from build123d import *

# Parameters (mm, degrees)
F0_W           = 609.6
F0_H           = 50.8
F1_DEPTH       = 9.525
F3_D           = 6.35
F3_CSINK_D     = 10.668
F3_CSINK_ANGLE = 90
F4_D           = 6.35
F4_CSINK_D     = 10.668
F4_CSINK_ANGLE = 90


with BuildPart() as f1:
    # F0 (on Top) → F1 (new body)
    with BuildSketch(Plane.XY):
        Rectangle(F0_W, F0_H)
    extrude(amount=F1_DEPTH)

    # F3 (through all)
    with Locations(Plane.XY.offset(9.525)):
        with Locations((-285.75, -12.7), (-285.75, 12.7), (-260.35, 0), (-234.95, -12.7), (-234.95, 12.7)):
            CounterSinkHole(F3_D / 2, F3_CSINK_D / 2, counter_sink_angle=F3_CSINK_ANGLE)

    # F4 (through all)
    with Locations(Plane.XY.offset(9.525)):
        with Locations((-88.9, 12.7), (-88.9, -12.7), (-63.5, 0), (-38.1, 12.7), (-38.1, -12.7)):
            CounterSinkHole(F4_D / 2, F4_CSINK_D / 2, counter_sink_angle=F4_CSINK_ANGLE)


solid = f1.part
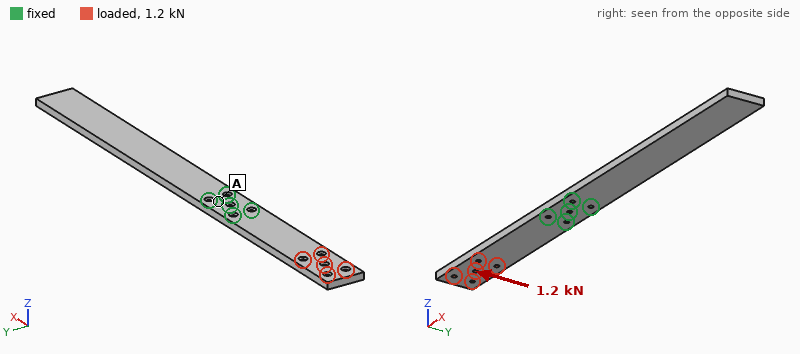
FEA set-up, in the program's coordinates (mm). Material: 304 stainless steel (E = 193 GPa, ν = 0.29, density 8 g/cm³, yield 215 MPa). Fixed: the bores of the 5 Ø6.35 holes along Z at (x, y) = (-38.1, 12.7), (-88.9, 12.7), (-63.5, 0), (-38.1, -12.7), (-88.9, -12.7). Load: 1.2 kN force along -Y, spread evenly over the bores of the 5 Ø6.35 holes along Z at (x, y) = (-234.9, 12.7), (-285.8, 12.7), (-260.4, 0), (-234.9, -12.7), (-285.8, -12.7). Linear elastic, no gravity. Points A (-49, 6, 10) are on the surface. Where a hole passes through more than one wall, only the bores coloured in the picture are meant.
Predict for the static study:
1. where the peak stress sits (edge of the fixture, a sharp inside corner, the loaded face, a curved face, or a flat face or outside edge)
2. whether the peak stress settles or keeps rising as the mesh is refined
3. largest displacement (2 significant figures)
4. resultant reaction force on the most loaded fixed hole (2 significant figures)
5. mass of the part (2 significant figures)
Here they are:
edge of the fixture
keeps rising
0.16 mm
5.6 kN
2.3 kg
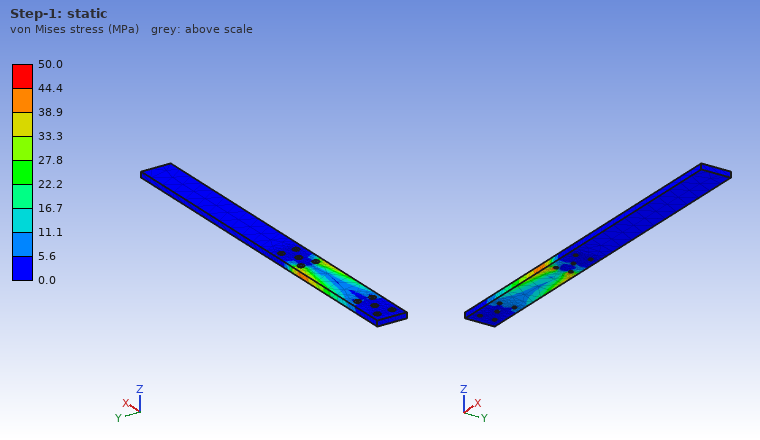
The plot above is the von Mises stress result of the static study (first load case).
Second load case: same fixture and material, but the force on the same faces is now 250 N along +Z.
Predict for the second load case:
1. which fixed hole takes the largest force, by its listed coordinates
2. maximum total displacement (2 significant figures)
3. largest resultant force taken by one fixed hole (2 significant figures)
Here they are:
(-63.5, 0)
0.85 mm
450 N
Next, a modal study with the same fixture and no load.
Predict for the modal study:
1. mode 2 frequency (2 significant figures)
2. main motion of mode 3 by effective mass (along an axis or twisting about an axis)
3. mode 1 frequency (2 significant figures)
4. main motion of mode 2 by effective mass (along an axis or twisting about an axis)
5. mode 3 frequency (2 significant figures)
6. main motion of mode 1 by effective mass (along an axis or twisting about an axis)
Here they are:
160 Hz
along Y
64 Hz
along Z
330 Hz
along Z
